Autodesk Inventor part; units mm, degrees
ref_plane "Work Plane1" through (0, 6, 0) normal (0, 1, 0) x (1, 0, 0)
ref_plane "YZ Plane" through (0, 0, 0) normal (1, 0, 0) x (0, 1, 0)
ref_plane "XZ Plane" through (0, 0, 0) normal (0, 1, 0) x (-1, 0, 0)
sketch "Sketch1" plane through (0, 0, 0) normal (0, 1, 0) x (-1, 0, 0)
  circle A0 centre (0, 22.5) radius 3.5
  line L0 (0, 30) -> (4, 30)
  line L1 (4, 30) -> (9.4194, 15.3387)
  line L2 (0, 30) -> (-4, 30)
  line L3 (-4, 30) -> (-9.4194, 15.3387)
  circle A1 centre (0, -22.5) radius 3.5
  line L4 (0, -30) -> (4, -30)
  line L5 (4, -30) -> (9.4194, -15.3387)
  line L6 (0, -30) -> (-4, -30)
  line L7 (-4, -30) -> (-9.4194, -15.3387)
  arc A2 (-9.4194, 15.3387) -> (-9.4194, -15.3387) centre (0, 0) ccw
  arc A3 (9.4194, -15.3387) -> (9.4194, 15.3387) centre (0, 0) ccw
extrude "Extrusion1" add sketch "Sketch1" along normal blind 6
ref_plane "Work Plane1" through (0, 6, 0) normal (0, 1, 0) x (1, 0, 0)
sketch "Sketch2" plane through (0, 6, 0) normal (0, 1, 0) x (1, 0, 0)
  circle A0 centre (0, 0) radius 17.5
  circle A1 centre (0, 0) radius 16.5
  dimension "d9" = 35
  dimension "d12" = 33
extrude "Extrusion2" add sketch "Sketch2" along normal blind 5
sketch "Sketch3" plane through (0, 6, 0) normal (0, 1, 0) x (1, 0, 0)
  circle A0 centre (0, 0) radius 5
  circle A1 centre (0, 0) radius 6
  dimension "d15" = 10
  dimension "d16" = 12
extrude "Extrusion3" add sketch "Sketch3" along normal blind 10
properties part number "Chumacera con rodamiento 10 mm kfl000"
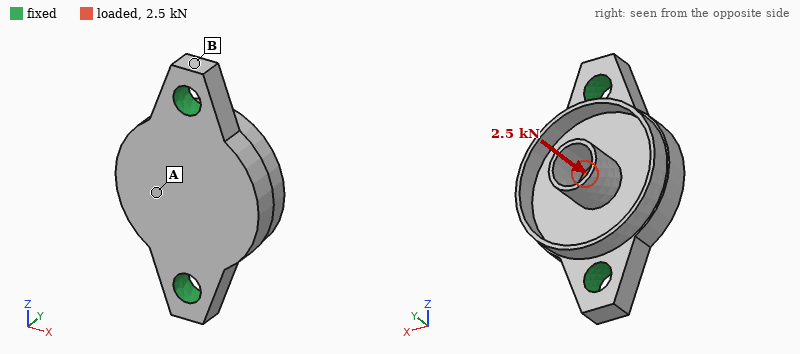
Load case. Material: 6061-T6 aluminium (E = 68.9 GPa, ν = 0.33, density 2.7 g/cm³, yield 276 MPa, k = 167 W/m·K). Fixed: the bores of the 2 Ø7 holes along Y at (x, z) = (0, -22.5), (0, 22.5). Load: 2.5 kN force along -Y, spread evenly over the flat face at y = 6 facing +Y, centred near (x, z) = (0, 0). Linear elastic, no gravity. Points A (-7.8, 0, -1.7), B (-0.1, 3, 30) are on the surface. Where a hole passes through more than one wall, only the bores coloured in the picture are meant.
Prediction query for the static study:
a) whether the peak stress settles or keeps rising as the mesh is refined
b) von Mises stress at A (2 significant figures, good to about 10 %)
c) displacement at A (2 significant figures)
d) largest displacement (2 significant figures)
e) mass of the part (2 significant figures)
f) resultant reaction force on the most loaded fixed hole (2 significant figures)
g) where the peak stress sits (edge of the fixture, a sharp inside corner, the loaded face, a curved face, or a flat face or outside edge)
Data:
keeps rising
47 MPa
31 µm
37 µm
23 g
1.3 kN
edge of the fixture
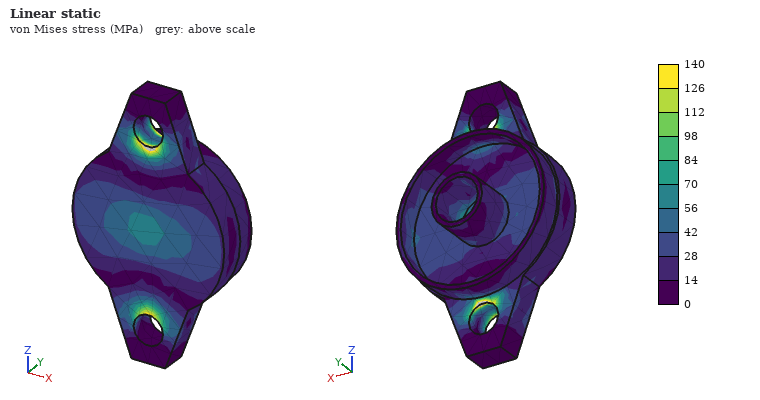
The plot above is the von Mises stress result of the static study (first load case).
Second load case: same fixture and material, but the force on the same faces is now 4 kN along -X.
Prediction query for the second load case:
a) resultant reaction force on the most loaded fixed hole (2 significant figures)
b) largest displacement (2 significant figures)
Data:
2.0 kN
43 µm
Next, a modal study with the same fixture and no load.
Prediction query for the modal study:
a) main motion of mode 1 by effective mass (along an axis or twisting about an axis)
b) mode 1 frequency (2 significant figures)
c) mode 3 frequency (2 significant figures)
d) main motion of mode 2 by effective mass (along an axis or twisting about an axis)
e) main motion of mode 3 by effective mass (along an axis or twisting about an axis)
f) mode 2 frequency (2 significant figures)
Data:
twisting about Z
9900 Hz
24 kHz
along Y
along X
12 kHz
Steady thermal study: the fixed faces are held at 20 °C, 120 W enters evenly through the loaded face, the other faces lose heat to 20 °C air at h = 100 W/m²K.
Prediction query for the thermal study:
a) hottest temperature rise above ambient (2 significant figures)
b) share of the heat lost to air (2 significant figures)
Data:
73 K
12 %
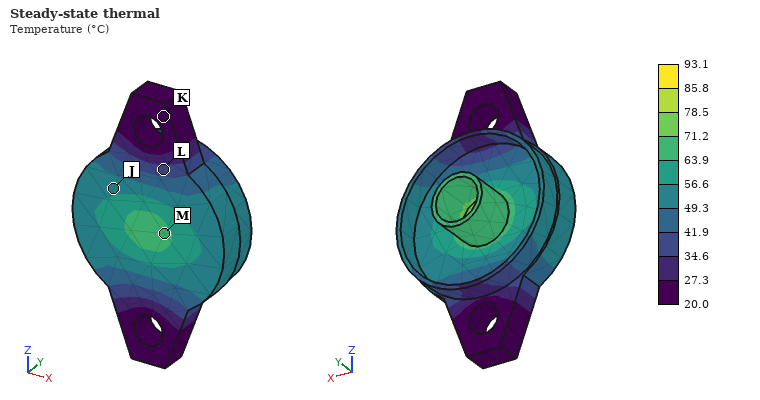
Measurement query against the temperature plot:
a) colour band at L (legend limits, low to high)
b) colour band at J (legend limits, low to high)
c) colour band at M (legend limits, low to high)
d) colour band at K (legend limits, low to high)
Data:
34.6 to 41.9 °C
49.3 to 56.6 °C
63.9 to 71.2 °C
20.0 to 27.3 °C
